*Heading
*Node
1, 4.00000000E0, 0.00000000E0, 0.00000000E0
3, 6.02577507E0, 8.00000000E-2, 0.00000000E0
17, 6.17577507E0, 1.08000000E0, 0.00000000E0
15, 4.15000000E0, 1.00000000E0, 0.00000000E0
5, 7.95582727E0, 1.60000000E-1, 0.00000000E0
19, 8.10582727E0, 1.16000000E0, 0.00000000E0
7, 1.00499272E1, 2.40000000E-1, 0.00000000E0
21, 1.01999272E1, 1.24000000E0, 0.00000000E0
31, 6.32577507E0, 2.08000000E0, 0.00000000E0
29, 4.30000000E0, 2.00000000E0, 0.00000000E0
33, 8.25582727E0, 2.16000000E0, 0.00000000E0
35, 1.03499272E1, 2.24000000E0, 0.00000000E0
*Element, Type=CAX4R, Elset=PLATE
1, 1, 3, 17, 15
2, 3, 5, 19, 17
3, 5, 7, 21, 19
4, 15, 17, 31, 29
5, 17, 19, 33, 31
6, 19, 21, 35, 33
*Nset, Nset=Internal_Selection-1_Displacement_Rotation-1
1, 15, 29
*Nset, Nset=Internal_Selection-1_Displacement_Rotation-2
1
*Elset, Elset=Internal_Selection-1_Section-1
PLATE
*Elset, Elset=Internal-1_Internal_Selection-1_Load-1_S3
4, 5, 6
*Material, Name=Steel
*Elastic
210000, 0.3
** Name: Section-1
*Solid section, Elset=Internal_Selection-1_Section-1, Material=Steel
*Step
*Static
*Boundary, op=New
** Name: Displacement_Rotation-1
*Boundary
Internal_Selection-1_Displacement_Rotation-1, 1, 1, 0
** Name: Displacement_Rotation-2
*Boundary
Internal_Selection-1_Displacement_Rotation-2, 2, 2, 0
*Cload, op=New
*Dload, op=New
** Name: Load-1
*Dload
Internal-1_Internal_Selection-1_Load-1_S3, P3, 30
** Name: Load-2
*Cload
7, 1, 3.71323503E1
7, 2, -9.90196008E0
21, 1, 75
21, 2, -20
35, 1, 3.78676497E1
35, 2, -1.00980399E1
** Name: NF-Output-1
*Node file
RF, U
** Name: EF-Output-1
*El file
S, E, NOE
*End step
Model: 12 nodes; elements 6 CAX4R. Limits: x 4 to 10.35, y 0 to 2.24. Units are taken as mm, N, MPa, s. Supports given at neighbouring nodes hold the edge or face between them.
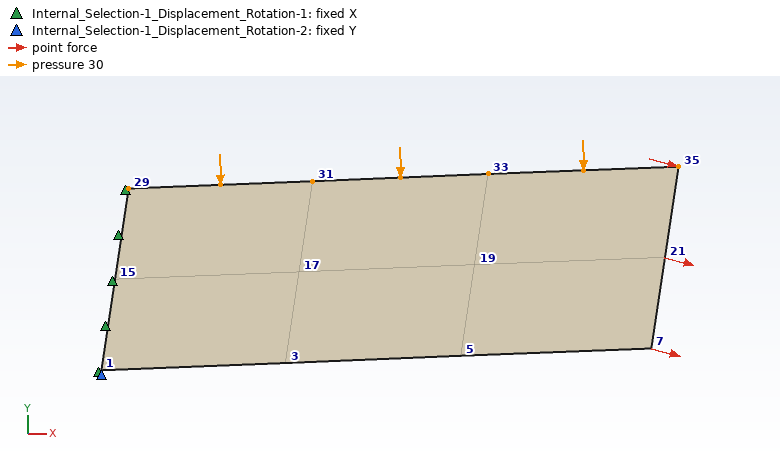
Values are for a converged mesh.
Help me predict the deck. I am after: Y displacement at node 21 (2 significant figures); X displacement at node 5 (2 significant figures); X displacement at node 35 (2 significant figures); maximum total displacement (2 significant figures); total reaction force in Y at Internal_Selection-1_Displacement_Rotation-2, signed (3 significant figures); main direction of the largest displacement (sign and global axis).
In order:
-0.048 mm
-0.0072 mm
0.0093 mm
0.050 mm
8390 N
-Y
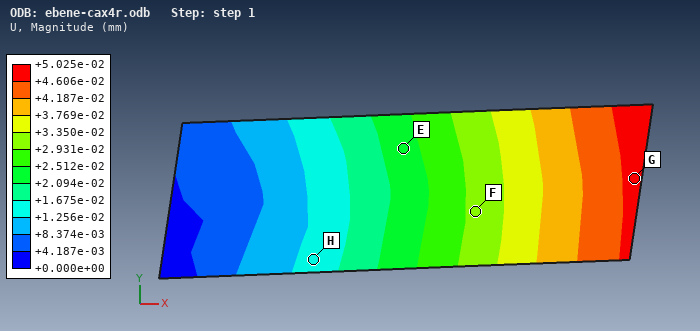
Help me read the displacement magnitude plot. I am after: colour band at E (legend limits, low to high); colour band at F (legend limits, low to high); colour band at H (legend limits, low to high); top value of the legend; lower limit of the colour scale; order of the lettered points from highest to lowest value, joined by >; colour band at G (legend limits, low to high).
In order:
+2.094e-02 to +2.512e-02 mm
+2.931e-02 to +3.350e-02 mm
+1.256e-02 to +1.675e-02 mm
+5.025e-02 mm
+0.000e+00 mm
G > F > E > H
+4.606e-02 to +5.025e-02 mm
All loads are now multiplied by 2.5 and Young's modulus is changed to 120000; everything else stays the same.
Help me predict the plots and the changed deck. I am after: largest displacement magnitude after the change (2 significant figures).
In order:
0.22 mm
